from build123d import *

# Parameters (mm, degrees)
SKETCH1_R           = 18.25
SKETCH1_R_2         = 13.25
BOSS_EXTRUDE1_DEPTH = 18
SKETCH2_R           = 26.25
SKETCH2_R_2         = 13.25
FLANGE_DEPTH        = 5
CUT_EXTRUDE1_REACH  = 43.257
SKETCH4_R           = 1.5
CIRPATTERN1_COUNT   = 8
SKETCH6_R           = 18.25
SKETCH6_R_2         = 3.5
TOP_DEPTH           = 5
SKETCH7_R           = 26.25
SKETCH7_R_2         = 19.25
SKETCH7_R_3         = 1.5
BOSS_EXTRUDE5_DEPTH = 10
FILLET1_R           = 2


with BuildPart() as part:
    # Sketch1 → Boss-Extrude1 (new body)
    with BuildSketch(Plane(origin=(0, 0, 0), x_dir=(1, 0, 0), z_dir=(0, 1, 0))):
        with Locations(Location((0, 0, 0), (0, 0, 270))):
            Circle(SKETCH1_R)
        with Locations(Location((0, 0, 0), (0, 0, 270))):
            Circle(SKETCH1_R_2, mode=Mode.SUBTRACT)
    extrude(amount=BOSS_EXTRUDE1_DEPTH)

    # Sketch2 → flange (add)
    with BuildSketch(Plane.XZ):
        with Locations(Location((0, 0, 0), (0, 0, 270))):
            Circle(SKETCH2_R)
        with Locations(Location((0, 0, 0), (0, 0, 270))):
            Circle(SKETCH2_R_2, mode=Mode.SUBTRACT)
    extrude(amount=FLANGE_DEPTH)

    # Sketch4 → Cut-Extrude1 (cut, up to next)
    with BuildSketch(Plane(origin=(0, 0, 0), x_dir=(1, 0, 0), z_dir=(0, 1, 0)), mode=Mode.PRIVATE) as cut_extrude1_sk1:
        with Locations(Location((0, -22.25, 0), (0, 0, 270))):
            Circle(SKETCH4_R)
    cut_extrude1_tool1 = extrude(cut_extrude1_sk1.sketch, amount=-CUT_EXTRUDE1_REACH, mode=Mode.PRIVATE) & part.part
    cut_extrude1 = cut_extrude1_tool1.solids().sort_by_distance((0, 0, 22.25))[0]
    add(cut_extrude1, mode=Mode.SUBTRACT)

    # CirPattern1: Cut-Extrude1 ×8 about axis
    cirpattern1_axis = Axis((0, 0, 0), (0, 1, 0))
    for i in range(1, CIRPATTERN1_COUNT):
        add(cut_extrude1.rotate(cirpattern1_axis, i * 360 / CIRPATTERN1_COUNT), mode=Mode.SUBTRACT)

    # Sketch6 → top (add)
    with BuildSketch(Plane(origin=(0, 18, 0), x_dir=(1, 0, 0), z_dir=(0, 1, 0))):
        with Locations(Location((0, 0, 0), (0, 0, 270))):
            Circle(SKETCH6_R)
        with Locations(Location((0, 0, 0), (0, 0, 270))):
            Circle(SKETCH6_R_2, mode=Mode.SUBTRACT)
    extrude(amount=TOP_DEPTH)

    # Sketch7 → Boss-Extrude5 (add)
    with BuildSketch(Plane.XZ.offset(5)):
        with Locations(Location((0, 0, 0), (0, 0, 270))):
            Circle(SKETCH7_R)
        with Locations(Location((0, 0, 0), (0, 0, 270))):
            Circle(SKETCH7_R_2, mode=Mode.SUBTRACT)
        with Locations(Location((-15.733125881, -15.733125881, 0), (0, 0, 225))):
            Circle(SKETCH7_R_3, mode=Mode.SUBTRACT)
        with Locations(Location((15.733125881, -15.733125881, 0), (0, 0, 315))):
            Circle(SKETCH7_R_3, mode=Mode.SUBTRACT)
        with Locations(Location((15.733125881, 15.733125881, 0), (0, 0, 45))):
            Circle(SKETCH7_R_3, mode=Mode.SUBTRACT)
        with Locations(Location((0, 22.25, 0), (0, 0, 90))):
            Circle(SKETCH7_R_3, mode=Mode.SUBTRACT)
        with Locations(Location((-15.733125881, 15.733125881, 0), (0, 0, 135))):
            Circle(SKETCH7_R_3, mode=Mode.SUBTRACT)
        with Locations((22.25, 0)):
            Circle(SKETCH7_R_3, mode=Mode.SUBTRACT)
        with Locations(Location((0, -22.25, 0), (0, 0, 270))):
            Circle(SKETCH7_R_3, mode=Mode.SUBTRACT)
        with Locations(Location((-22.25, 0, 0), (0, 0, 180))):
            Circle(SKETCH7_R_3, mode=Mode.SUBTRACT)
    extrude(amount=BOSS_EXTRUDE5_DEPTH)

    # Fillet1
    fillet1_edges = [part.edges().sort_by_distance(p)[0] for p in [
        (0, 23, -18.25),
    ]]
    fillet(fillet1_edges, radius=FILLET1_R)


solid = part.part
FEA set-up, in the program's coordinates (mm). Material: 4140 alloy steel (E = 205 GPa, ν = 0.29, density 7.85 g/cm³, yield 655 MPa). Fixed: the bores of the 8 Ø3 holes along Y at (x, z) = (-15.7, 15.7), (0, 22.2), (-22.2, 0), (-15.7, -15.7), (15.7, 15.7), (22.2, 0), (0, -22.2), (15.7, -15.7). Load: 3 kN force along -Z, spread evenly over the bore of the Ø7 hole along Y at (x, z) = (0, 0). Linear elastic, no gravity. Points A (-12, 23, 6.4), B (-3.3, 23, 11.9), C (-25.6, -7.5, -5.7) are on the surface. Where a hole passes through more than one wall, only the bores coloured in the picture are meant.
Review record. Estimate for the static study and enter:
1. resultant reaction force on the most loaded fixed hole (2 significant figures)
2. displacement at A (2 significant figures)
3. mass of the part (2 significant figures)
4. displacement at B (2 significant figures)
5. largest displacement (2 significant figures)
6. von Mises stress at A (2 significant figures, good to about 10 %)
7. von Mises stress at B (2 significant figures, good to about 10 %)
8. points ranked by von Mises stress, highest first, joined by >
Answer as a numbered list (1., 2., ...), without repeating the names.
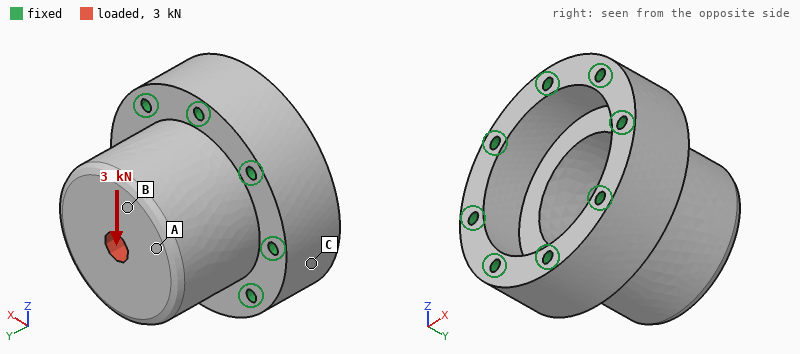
1. 1.0 kN
2. 5.3 µm
3. 240 g
4. 6.2 µm
5. 6.8 µm
6. 8.4 MPa
7. 17 MPa
8. B > A > C
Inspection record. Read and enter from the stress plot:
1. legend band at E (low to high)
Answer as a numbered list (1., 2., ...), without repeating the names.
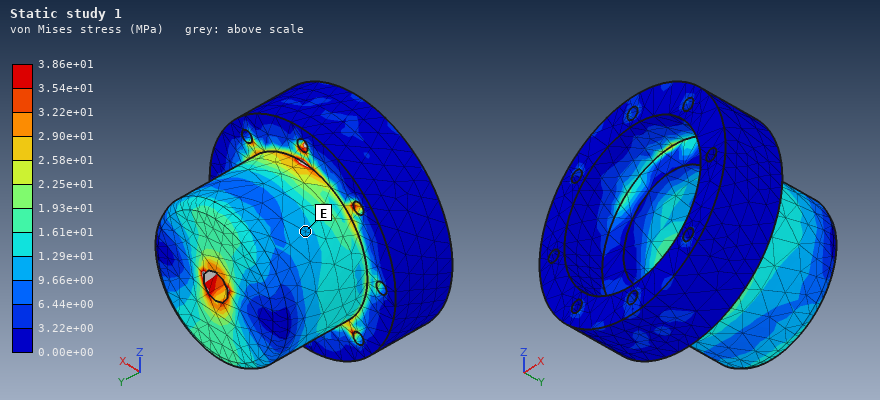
1. 9.66e+00 to 1.29e+01 MPa
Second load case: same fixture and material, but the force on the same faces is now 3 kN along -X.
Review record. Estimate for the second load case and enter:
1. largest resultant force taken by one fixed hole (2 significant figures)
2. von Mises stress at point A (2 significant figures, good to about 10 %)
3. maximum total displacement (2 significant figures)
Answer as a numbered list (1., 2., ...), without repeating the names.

1. 1.0 kN
2. 16 MPa
3. 6.8 µm
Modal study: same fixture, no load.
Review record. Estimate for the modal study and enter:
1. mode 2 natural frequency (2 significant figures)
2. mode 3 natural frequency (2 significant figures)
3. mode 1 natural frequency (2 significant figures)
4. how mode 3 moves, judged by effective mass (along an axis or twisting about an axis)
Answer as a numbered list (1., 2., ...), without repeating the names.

1. 16 kHz
2. 26 kHz
3. 16 kHz
4. along Y
